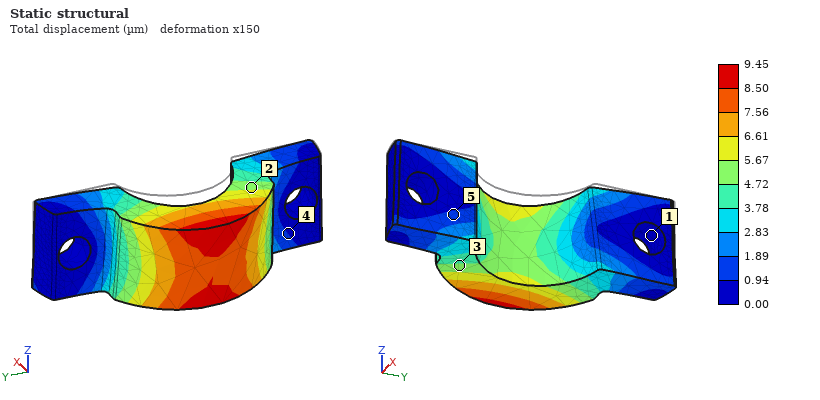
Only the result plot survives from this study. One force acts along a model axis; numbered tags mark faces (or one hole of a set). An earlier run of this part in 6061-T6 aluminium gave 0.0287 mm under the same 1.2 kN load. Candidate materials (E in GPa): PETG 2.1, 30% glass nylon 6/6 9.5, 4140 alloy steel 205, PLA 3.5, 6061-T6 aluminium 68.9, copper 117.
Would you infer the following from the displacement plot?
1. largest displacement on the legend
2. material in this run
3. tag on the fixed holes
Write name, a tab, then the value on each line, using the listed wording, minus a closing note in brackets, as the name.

largest displacement on the legend	9.45 µm
material in this run	4140 alloy steel
tag on the fixed holes	1
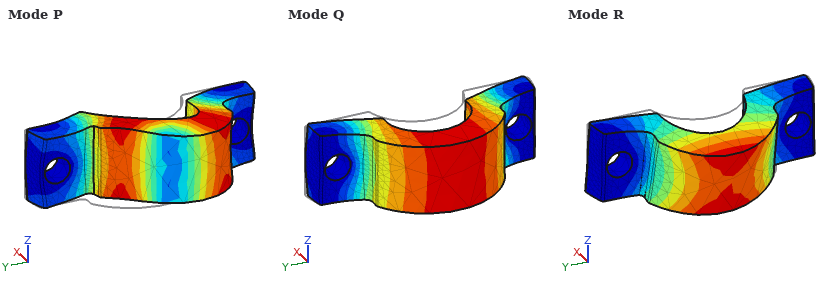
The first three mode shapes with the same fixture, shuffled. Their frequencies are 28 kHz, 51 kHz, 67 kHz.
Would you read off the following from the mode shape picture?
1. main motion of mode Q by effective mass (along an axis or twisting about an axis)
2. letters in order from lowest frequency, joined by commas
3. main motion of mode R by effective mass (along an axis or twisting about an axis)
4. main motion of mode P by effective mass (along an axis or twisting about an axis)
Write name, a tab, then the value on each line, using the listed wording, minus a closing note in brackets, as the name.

main motion of mode Q by effective mass	along X
letters in order from lowest frequency, joined by commas	R, Q, P
main motion of mode R by effective mass	along Z
main motion of mode P by effective mass	along Y
